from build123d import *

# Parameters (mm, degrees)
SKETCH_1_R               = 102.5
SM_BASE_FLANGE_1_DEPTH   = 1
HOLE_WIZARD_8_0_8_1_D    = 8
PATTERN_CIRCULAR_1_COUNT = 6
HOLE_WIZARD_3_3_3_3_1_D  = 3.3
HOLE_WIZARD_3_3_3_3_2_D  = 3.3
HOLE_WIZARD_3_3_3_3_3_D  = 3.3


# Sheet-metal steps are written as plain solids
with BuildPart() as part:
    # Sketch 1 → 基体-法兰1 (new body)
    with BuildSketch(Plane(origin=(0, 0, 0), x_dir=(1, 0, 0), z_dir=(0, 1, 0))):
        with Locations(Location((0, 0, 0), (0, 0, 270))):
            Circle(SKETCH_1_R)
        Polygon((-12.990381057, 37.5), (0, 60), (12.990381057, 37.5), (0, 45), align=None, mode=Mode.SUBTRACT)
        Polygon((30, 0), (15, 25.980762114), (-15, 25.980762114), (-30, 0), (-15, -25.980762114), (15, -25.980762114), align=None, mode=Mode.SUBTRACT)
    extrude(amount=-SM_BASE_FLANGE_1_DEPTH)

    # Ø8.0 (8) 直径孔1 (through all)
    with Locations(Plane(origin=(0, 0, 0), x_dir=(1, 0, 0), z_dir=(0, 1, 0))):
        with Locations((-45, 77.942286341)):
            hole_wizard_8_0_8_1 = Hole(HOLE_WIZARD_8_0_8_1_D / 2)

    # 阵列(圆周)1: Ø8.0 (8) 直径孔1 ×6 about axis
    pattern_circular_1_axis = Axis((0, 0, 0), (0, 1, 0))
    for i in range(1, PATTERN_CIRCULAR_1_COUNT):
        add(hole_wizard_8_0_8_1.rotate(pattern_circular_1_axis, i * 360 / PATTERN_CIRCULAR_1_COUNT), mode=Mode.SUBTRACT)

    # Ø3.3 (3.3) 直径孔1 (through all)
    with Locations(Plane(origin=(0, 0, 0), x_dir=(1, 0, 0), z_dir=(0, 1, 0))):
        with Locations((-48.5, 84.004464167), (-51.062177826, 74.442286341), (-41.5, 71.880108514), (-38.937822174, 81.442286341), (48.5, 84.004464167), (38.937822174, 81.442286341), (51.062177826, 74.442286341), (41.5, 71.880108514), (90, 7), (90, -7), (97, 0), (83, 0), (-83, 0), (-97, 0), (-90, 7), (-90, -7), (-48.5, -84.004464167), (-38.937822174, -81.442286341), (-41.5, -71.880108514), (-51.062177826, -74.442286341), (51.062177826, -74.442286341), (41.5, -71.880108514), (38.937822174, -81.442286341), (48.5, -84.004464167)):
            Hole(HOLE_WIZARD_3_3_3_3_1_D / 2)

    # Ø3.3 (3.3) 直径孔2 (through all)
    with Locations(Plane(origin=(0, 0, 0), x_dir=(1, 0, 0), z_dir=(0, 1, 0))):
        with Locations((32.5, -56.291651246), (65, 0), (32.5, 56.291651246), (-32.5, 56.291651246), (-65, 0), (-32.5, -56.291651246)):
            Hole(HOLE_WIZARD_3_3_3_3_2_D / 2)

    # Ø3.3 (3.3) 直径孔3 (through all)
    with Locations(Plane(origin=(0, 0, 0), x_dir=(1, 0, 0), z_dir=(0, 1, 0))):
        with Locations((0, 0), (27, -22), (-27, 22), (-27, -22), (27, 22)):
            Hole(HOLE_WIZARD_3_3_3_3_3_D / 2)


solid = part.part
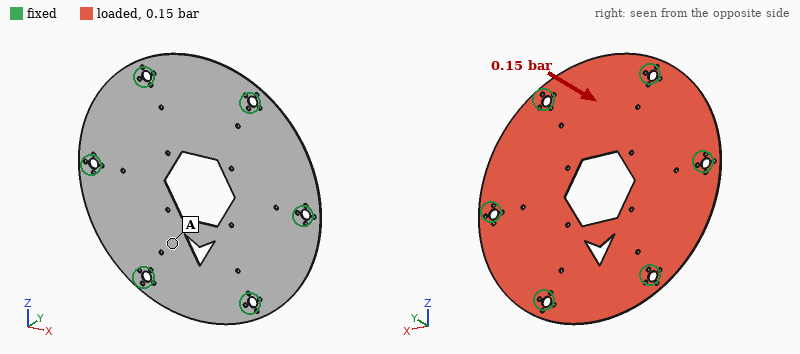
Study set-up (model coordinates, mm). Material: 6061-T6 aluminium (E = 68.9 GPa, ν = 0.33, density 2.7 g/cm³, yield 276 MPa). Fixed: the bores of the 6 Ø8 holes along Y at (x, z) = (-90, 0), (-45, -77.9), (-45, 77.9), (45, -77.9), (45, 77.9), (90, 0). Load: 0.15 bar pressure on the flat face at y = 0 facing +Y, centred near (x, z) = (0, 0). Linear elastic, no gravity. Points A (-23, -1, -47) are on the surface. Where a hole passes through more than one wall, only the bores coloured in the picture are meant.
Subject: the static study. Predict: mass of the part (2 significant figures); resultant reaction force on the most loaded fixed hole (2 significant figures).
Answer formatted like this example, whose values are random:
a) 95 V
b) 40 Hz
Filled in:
a) 81 g
b) 75 N
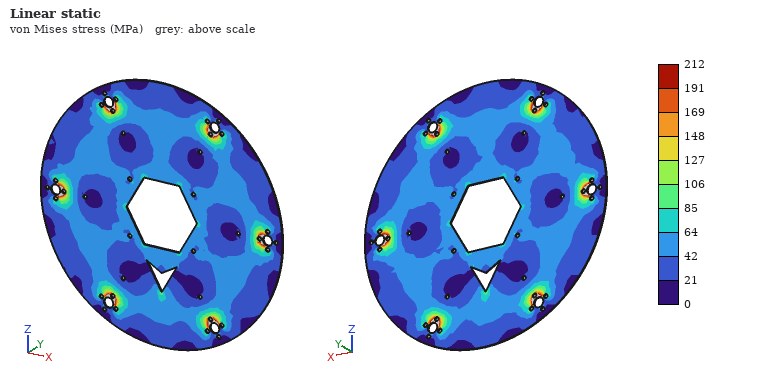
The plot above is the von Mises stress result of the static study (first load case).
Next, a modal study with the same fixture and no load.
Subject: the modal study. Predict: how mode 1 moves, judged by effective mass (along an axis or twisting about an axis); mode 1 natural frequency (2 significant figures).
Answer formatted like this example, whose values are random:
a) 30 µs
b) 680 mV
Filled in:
a) along Y
b) 280 Hz
